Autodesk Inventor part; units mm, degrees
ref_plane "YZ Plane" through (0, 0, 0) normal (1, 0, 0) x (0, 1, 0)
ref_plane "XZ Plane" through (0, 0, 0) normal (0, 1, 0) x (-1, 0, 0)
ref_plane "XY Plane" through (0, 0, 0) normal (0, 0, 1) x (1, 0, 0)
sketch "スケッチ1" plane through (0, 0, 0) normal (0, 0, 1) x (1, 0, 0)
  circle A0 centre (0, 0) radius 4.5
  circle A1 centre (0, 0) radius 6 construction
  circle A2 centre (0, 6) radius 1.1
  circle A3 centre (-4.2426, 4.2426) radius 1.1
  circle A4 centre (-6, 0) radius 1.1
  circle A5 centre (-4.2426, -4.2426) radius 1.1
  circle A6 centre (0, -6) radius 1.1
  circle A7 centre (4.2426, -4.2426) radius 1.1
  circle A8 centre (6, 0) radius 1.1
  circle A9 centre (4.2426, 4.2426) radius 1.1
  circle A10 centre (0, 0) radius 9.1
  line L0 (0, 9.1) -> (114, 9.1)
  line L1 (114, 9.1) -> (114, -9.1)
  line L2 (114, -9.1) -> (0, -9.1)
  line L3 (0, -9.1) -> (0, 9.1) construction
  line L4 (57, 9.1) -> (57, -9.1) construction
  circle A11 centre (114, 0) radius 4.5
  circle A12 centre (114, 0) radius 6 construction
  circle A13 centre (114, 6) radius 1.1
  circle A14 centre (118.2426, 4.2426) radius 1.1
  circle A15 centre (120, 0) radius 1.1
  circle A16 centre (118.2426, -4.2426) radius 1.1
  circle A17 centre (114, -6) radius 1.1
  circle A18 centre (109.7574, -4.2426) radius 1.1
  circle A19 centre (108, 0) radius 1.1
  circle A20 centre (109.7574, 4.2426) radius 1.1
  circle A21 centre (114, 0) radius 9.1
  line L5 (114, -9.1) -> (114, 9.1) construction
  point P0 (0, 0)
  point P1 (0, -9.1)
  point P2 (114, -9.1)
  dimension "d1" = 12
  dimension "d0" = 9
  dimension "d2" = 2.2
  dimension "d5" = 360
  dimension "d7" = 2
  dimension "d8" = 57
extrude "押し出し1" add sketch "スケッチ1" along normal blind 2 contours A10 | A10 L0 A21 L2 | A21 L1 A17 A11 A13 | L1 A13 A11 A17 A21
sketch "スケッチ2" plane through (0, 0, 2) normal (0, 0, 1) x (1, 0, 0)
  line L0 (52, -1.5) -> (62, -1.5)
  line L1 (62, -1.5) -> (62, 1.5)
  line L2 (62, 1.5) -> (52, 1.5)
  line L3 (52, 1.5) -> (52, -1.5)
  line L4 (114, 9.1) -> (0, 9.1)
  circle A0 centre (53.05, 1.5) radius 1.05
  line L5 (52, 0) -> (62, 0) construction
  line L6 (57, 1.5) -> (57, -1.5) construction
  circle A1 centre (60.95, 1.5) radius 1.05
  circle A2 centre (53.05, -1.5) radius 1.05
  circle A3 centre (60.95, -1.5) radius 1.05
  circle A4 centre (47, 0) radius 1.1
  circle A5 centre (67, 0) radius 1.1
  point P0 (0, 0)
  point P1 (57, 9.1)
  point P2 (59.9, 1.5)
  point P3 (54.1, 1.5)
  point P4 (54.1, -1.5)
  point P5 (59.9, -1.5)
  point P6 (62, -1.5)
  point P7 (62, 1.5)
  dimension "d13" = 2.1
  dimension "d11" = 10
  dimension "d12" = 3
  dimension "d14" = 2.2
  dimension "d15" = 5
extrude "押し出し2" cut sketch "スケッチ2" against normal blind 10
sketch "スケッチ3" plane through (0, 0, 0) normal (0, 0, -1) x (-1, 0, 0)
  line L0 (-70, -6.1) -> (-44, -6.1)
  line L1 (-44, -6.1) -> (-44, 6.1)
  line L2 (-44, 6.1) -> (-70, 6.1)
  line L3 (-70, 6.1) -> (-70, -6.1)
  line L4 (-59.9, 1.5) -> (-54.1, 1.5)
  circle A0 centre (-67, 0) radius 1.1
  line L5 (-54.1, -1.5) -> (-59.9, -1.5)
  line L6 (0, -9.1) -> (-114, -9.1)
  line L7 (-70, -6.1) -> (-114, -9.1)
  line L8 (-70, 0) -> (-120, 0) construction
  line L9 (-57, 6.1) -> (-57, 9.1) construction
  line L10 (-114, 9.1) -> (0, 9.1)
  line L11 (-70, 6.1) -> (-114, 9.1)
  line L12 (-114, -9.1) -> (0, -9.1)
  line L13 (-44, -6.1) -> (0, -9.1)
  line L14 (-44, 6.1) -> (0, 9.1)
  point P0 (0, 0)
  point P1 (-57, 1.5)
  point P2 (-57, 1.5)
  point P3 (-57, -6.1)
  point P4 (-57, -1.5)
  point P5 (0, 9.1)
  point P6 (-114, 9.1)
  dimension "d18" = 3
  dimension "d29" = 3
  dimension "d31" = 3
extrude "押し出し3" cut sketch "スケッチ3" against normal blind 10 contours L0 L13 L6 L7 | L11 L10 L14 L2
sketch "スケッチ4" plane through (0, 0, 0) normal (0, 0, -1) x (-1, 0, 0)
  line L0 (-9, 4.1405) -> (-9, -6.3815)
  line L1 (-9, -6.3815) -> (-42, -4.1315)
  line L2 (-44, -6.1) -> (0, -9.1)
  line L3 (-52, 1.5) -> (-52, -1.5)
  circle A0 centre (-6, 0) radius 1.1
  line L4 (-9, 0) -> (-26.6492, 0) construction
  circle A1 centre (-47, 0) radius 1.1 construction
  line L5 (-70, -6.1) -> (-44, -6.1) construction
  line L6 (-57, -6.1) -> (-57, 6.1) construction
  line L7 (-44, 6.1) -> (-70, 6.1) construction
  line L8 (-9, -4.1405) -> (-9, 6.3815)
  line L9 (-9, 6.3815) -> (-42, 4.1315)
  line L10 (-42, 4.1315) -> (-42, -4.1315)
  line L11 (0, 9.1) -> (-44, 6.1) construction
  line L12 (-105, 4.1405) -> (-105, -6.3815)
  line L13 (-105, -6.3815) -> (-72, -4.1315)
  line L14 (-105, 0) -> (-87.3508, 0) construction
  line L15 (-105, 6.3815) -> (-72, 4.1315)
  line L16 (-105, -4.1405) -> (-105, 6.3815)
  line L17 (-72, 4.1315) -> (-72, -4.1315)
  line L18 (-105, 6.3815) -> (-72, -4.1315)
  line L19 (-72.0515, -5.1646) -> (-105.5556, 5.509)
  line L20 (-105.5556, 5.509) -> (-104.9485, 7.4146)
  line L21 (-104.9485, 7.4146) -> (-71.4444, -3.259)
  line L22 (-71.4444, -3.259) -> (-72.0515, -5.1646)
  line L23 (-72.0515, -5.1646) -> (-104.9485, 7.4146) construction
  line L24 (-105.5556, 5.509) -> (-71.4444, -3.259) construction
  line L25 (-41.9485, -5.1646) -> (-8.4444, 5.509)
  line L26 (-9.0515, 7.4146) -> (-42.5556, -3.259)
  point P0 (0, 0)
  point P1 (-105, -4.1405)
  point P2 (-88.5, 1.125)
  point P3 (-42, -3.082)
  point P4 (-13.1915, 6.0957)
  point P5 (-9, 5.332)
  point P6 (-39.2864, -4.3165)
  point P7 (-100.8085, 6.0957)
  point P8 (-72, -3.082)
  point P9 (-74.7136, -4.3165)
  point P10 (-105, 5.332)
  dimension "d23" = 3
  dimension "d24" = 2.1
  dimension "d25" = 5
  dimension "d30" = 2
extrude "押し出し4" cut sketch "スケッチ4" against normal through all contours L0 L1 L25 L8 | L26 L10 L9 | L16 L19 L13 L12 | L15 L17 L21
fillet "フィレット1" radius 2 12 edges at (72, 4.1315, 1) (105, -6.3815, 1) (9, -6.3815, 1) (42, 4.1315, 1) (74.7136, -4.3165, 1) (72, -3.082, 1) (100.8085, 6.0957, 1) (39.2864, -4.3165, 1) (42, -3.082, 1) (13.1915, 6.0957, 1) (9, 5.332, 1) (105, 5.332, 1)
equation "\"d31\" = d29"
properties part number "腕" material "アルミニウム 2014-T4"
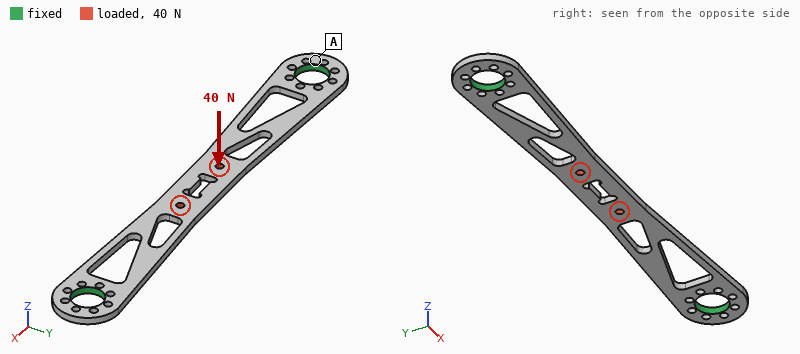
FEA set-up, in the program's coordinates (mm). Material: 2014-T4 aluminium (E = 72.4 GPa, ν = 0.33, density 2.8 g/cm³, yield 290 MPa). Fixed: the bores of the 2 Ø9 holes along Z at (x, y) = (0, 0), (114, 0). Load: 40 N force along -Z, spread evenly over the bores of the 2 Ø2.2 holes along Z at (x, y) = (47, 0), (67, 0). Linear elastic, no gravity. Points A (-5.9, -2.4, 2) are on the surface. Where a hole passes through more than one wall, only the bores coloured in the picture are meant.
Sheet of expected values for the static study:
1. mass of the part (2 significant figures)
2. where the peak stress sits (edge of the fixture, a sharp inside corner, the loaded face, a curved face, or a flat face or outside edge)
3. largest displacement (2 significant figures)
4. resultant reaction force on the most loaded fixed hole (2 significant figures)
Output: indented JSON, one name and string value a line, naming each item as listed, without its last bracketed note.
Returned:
{
  "mass of the part": "6.8 g",
  "where the peak stress sits": "a curved face",
  "largest displacement": "0.58 mm",
  "resultant reaction force on the most loaded fixed hole": "20 N"
}
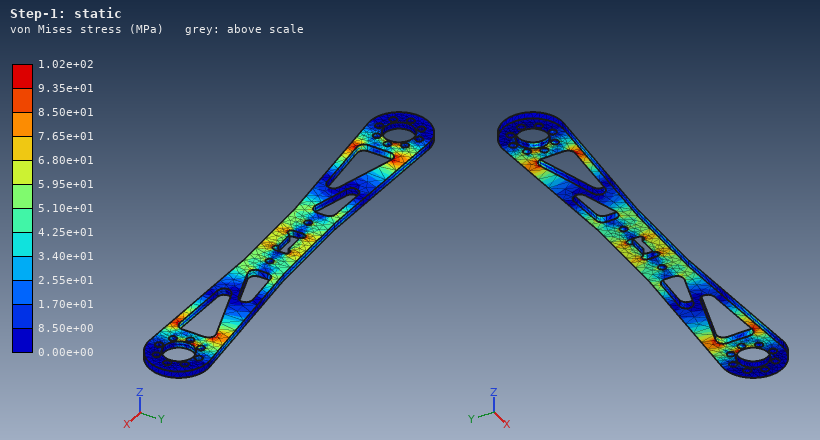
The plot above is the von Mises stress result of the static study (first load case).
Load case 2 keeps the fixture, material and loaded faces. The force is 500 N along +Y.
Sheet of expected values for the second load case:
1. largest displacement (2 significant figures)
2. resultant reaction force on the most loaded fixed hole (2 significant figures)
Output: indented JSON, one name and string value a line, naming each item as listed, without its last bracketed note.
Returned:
{
  "largest displacement": "0.25 mm",
  "resultant reaction force on the most loaded fixed hole": "300 N"
}
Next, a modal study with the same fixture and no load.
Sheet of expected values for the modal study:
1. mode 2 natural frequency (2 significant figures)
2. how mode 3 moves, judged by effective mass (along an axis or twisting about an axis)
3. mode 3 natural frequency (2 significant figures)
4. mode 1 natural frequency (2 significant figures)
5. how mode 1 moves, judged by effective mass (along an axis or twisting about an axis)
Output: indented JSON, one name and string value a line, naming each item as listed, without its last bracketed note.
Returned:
{
  "mode 2 natural frequency": "2400 Hz",
  "how mode 3 moves, judged by effective mass": "twisting about X",
  "mode 3 natural frequency": "3300 Hz",
  "mode 1 natural frequency": "850 Hz",
  "how mode 1 moves, judged by effective mass": "along Z"
}
